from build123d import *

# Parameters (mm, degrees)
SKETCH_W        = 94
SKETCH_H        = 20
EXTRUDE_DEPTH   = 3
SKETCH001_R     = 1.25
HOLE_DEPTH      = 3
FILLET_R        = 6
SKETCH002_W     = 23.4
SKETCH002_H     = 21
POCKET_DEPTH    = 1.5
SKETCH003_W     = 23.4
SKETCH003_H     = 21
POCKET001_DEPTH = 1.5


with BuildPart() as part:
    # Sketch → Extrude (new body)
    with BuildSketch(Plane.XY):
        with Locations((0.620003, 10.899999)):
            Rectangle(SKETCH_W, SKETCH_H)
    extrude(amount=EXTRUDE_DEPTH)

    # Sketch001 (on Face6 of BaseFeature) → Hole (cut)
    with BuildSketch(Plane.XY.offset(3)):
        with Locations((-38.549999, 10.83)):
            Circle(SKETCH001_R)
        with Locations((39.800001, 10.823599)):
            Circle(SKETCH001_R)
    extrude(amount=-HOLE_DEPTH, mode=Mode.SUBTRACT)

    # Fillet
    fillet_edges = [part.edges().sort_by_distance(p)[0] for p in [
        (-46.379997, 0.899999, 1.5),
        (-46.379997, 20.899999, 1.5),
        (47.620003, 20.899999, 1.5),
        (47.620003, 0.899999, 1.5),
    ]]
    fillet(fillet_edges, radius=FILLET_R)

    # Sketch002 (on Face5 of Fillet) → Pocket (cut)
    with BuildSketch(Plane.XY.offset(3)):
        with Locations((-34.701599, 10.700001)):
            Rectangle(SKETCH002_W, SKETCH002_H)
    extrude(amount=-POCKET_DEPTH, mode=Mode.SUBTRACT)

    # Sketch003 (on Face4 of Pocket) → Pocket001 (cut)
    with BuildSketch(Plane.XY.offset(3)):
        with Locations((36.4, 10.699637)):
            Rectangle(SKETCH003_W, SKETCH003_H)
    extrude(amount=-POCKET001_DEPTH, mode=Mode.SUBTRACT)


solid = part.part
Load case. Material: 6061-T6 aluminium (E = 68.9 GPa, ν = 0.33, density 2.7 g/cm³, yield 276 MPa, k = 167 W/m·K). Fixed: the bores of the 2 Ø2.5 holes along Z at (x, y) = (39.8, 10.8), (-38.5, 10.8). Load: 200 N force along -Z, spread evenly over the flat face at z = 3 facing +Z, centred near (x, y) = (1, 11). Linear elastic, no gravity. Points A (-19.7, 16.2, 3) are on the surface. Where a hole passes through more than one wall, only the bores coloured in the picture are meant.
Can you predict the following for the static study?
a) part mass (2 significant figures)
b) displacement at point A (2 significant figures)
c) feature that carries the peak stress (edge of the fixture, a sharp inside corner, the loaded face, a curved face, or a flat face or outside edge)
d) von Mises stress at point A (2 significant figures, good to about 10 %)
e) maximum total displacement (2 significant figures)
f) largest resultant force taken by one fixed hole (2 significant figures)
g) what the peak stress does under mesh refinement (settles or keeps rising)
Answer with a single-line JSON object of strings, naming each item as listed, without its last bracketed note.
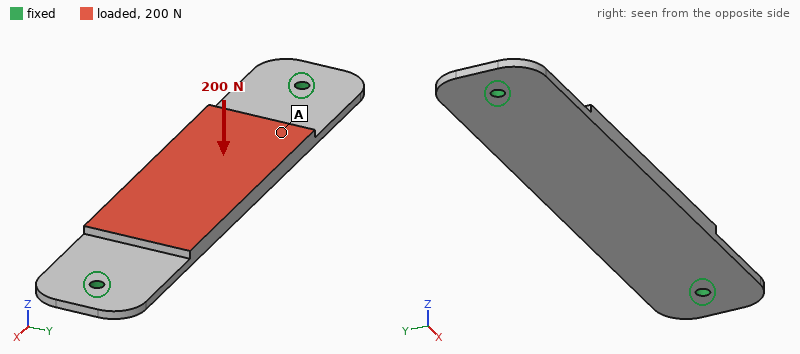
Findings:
{"part mass": "11 g", "displacement at point A": "0.19 mm", "feature that carries the peak stress": "edge of the fixture", "von Mises stress at point A": "28 MPa", "maximum total displacement": "0.29 mm", "largest resultant force taken by one fixed hole": "380 N", "what the peak stress does under mesh refinement": "keeps rising"}
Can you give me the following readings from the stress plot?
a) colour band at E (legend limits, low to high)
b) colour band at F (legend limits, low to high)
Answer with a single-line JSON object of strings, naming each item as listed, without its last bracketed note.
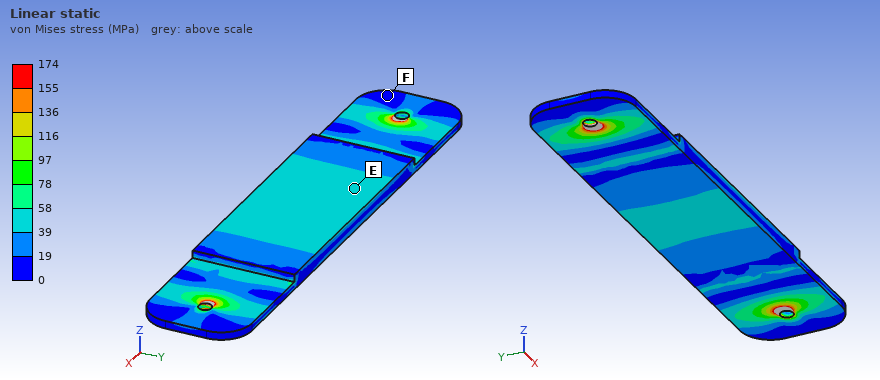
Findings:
{"colour band at E": "39 to 58 MPa", "colour band at F": "0 to 19 MPa"}
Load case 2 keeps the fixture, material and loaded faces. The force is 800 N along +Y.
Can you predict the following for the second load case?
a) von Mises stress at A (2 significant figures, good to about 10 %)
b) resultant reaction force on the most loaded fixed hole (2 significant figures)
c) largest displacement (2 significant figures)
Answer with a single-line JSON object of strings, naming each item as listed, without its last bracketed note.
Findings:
{"von Mises stress at A": "50 MPa", "resultant reaction force on the most loaded fixed hole": "400 N", "largest displacement": "0.27 mm"}
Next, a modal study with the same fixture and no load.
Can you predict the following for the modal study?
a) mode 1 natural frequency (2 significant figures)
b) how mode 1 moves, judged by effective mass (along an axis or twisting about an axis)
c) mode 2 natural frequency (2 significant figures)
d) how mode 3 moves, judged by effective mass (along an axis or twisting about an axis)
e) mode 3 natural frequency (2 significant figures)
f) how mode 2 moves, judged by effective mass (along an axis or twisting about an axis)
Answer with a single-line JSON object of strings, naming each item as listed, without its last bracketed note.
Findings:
{"mode 1 natural frequency": "1600 Hz", "how mode 1 moves, judged by effective mass": "along Z", "mode 2 natural frequency": "2600 Hz", "how mode 3 moves, judged by effective mass": "twisting about Y", "mode 3 natural frequency": "4200 Hz", "how mode 2 moves, judged by effective mass": "twisting about X"}
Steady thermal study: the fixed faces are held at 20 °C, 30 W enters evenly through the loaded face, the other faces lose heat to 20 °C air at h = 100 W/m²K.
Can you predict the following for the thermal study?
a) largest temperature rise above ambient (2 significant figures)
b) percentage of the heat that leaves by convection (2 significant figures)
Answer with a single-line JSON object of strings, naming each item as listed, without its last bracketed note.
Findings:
{"largest temperature rise above ambient": "54 K", "percentage of the heat that leaves by convection": "32 %"}
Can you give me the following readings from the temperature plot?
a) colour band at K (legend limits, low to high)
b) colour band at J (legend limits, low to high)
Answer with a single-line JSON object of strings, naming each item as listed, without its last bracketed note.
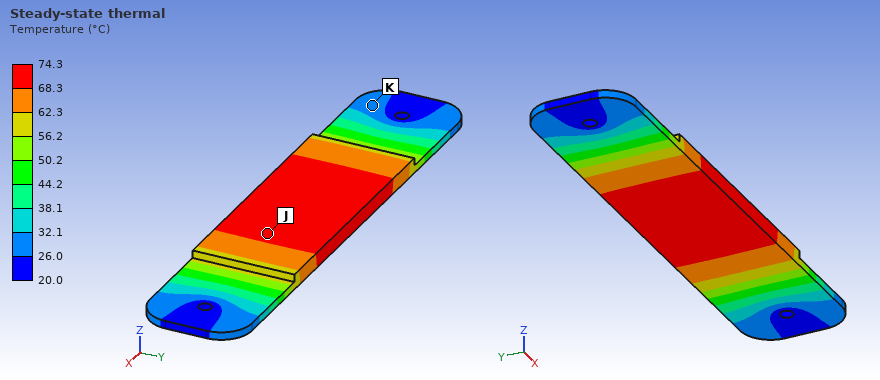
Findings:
{"colour band at K": "26.0 to 32.1 °C", "colour band at J": "68.3 to 74.3 °C"}
